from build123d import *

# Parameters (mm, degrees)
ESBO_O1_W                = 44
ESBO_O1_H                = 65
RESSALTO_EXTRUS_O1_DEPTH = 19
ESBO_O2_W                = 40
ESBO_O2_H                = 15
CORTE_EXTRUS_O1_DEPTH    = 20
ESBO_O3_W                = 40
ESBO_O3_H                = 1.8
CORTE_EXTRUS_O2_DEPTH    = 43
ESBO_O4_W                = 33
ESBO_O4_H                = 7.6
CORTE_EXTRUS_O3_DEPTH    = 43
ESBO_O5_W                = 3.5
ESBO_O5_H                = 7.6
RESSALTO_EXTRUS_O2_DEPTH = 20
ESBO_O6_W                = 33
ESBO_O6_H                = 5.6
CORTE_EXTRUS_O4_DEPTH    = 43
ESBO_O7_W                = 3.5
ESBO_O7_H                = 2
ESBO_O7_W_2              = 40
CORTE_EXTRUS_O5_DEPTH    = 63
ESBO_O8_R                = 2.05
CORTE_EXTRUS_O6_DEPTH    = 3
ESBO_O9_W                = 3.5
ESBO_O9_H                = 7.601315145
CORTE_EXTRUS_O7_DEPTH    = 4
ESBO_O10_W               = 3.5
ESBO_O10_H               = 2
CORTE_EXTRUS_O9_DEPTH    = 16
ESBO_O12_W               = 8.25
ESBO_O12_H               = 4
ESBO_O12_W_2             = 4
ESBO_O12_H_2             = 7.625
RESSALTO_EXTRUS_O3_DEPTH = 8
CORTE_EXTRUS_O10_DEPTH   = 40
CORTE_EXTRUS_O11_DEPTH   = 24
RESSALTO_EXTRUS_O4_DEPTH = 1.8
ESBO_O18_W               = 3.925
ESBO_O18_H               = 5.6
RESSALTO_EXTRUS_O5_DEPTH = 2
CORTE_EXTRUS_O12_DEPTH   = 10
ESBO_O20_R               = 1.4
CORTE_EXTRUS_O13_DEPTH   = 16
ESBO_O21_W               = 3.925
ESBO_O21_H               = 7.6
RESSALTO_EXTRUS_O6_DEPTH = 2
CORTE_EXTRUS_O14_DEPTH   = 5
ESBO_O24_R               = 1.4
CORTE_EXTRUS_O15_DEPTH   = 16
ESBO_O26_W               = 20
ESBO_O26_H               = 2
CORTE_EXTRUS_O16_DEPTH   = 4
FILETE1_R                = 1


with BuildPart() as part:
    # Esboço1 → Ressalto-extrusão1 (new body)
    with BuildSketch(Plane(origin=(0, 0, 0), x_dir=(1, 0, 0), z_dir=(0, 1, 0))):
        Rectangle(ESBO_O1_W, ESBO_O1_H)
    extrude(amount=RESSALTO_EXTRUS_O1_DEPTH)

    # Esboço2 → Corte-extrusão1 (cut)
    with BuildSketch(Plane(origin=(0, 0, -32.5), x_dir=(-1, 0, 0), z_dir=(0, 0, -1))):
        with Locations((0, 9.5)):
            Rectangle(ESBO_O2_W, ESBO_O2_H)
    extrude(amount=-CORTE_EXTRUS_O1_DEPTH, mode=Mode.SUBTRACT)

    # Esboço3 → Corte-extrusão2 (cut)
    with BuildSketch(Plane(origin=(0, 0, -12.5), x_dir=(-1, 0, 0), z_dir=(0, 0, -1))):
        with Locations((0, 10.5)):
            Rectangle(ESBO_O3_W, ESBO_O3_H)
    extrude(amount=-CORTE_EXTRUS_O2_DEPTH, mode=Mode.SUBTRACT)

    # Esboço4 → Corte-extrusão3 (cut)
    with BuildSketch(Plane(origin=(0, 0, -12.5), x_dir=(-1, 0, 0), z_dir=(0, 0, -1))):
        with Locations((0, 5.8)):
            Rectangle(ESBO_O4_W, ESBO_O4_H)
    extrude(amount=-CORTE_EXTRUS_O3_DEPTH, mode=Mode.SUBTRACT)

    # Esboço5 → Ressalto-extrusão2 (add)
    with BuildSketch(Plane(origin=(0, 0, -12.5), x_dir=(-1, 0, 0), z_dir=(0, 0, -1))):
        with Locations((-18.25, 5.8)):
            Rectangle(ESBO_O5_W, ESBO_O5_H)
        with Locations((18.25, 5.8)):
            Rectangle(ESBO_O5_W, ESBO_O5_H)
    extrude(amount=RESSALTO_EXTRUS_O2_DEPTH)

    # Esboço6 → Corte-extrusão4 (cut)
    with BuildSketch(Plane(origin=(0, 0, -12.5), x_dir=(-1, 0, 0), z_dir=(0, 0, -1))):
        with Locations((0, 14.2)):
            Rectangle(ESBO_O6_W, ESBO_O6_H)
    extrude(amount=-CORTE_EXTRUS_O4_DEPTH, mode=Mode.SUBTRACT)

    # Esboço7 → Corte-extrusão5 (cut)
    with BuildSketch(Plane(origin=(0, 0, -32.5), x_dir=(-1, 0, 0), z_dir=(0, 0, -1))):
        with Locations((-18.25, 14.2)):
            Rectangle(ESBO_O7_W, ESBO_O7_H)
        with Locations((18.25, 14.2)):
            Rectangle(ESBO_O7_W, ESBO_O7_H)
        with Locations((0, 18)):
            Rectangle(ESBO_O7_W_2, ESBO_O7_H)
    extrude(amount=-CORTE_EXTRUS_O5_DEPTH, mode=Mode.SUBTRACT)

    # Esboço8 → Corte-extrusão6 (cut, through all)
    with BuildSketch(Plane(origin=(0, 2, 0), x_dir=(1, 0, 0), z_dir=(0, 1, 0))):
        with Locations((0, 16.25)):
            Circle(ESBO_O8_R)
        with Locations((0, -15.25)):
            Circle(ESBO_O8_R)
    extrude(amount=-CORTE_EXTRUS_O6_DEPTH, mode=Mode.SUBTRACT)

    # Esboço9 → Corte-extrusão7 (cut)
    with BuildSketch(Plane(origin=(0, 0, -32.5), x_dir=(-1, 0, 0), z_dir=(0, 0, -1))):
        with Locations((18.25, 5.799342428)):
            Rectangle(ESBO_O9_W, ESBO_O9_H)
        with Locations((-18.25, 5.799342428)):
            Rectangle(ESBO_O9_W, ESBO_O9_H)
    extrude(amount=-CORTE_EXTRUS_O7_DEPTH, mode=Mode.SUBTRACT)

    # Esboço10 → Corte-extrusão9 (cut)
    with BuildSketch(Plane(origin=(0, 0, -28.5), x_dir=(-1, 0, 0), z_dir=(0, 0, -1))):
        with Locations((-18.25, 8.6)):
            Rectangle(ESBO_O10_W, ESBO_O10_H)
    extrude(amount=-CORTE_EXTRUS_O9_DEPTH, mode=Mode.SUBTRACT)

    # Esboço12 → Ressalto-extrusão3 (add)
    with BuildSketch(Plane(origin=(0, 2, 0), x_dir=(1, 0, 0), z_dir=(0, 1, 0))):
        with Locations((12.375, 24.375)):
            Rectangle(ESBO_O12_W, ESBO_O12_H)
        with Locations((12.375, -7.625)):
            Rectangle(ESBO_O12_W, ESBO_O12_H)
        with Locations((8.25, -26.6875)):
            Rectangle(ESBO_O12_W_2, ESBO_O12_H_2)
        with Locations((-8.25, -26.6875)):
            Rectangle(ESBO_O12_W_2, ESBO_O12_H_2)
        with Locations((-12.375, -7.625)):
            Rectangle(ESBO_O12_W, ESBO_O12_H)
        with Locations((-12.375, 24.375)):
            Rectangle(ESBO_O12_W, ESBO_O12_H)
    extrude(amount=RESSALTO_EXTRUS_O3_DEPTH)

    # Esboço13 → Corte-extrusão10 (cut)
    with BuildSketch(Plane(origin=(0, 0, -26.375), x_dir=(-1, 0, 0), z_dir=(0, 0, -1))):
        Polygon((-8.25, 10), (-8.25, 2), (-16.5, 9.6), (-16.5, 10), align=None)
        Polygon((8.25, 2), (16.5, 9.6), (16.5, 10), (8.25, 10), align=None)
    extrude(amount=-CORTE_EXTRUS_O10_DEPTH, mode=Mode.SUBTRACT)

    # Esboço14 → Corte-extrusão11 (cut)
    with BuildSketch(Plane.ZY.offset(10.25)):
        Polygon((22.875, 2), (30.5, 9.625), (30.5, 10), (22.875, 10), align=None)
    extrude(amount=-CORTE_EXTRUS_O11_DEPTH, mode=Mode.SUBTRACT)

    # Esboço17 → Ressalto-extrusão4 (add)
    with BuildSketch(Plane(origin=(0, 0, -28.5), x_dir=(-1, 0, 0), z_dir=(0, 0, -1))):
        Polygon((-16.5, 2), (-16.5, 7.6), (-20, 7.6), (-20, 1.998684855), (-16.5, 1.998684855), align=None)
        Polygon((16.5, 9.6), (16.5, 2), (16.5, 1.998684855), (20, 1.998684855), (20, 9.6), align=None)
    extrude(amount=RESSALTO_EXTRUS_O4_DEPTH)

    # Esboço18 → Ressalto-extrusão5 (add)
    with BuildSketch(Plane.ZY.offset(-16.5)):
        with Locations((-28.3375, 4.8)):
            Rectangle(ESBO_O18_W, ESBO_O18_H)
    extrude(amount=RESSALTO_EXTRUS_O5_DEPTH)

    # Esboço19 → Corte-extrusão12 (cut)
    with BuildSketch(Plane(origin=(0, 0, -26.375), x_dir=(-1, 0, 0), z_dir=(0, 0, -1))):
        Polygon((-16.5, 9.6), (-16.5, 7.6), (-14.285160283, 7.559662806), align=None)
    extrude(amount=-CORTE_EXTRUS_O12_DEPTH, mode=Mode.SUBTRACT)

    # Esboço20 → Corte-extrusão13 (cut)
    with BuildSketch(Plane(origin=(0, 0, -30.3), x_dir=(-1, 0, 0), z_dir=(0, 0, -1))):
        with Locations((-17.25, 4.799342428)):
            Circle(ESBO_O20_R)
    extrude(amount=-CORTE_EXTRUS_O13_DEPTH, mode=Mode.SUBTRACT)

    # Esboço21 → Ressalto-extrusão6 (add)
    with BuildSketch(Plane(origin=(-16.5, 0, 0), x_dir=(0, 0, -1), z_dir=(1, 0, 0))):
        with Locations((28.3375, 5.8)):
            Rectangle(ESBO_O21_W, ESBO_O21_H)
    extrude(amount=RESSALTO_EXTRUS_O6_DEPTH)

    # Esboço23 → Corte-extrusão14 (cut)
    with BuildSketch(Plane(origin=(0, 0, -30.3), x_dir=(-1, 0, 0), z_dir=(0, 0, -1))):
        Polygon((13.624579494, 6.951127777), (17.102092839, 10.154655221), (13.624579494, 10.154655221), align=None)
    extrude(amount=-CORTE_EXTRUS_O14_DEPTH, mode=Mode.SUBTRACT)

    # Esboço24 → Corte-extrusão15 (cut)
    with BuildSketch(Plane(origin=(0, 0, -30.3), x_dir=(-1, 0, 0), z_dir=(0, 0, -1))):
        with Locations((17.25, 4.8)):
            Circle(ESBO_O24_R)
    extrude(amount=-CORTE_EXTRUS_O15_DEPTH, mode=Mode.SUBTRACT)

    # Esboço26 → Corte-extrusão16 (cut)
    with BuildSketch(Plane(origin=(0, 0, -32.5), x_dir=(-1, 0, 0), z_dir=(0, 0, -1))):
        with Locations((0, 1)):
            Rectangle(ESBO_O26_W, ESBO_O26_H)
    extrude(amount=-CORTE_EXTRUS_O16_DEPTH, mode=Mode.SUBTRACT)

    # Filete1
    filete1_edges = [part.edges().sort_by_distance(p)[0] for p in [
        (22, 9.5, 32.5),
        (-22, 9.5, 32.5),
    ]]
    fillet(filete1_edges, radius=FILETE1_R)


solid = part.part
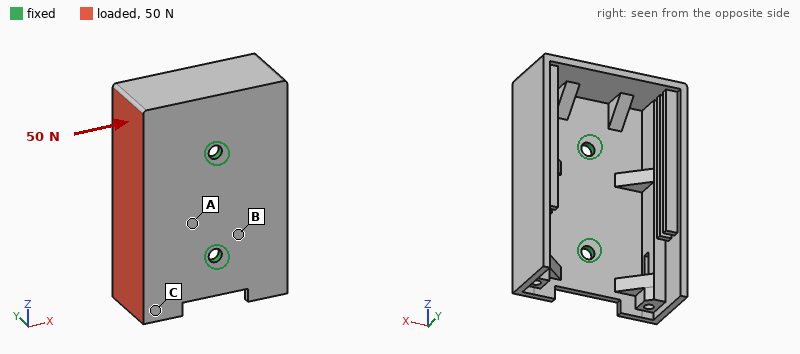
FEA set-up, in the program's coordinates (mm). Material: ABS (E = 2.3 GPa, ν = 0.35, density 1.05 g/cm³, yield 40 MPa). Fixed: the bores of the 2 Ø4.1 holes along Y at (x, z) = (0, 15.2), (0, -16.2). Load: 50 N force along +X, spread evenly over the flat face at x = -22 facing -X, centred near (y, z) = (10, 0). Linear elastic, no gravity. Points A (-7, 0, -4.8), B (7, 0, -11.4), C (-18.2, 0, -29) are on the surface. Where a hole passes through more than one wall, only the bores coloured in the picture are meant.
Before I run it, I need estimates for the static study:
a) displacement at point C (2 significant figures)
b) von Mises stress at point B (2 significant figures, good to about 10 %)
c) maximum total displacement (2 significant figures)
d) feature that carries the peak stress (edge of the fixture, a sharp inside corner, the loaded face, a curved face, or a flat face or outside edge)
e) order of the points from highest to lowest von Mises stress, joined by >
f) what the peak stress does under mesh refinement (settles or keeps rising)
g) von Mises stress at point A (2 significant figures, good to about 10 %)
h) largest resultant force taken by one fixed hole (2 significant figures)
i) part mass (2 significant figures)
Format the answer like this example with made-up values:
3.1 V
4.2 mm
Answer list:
0.41 mm
1.9 MPa
0.85 mm
edge of the fixture
A > B > C
keeps rising
3.5 MPa
25 N
17 g
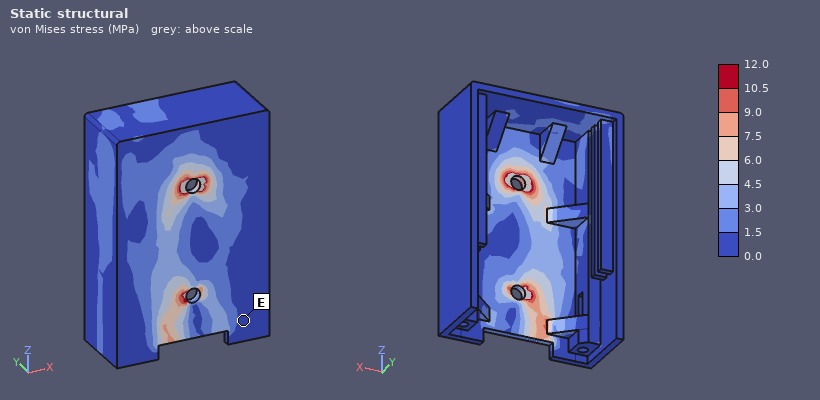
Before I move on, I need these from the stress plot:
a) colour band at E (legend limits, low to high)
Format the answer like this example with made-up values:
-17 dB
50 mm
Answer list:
0.0 to 1.5 MPa
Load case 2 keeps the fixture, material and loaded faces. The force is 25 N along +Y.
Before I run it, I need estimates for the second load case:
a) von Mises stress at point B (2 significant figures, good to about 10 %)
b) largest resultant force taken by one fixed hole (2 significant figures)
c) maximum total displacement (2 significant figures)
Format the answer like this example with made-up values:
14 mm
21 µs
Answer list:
2.1 MPa
13 N
0.88 mm
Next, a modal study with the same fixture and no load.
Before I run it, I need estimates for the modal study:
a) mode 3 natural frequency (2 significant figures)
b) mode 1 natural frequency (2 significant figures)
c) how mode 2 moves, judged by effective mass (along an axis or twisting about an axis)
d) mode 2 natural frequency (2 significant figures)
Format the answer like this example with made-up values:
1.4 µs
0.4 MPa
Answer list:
800 Hz
340 Hz
along Y
620 Hz
